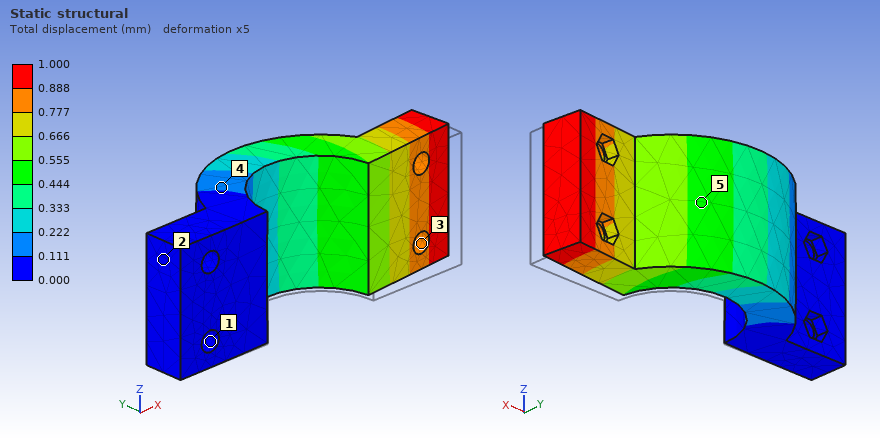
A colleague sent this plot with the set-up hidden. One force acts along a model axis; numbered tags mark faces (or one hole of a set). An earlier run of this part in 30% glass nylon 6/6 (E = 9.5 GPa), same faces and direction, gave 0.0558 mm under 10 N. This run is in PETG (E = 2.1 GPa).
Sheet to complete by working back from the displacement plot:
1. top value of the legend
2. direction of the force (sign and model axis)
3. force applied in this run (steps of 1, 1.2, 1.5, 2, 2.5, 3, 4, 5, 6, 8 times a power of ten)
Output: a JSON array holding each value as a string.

["1.000 mm", "+Y", "40 N"]
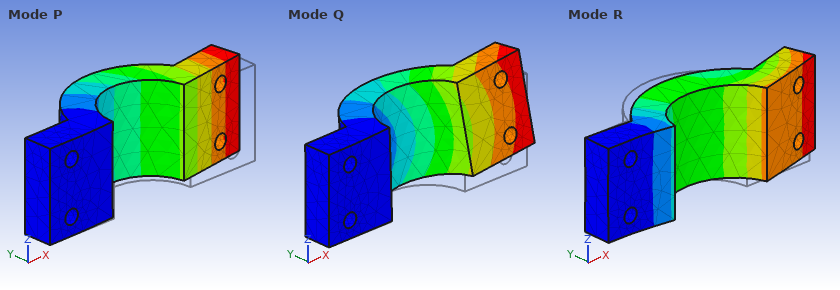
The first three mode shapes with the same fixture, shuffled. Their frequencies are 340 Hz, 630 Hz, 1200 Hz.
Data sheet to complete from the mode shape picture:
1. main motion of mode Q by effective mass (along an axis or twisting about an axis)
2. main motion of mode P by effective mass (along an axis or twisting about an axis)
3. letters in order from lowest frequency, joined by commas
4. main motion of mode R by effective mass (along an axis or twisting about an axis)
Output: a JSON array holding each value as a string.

["along Z", "along Y", "P, Q, R", "along X"]
